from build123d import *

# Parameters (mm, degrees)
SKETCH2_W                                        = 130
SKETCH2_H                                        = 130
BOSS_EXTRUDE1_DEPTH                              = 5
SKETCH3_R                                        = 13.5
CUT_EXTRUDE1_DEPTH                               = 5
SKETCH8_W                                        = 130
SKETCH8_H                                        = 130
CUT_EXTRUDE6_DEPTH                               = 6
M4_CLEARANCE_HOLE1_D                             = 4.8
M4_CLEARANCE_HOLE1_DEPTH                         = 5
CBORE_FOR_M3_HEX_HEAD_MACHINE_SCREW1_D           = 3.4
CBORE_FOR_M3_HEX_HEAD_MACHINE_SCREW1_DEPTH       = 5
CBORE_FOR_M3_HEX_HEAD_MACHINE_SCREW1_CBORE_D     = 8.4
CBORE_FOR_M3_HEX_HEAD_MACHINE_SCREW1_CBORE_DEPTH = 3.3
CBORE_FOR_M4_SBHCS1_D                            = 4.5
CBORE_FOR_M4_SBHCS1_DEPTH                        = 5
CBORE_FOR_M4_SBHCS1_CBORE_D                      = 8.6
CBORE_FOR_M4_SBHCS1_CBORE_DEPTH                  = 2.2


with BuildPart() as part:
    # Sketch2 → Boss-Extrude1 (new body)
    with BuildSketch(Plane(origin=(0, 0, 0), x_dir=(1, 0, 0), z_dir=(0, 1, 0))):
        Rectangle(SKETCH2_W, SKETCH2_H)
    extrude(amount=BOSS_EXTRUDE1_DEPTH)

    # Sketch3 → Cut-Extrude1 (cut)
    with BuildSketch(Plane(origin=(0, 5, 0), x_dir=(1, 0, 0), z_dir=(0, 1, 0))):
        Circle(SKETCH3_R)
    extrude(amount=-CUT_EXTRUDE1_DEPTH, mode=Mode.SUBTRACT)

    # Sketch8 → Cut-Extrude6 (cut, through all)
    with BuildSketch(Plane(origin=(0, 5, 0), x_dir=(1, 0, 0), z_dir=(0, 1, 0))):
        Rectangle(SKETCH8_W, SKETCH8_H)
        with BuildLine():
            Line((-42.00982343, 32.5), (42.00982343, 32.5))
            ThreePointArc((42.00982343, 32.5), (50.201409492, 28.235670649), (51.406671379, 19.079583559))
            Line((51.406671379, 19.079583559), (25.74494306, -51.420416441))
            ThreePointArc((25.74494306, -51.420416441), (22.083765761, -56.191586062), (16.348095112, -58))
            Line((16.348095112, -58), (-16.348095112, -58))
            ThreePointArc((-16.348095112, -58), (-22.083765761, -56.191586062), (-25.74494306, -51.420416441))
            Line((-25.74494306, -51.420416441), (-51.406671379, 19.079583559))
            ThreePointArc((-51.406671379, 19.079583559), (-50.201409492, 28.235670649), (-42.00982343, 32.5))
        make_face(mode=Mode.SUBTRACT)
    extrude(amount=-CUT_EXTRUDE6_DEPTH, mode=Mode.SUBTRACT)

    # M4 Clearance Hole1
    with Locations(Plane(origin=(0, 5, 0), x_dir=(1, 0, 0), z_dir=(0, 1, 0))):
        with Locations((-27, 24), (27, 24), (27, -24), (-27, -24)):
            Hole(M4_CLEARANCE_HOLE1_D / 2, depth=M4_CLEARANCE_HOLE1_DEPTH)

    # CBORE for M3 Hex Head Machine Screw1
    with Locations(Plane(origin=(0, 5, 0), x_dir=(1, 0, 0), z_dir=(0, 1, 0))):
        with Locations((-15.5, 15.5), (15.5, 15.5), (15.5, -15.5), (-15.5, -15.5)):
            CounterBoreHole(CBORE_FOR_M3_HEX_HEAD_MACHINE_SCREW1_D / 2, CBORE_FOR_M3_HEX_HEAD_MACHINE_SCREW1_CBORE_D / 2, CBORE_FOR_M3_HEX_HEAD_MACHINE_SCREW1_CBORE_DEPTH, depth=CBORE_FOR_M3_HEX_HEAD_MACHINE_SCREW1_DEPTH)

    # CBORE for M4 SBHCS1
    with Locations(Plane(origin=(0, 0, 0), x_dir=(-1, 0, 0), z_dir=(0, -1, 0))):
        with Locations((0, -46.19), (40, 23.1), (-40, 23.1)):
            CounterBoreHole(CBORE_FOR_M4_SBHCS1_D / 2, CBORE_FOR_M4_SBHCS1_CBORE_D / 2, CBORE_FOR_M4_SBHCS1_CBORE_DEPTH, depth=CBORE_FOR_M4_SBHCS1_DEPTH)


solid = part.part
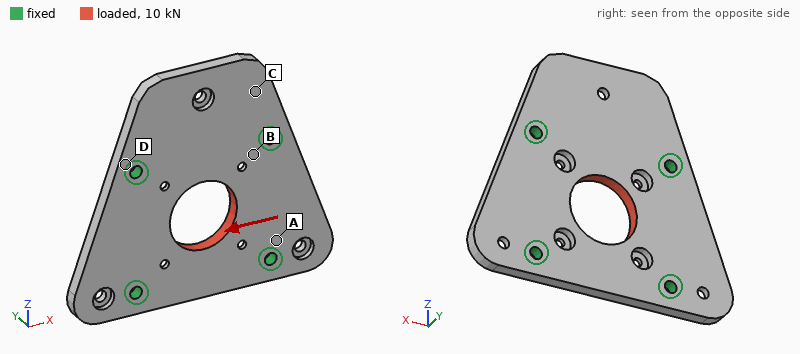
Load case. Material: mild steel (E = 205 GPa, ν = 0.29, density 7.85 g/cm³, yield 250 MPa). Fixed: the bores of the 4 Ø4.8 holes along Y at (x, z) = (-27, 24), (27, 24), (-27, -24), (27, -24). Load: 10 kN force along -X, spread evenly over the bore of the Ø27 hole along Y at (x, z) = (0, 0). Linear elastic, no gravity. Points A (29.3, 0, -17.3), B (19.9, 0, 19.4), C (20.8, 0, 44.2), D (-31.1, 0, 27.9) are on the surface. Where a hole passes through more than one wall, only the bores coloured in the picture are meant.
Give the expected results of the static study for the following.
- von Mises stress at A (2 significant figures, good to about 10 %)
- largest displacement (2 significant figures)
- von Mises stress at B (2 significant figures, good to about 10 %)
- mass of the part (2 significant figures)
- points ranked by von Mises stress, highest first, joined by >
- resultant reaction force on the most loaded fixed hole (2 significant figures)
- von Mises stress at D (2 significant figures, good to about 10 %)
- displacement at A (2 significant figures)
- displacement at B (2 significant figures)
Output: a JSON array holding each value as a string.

["23 MPa", "5.0 µm", "32 MPa", "240 g", "B > A > D > C", "2.6 kN", "12 MPa", "1.5 µm", "1.4 µm"]
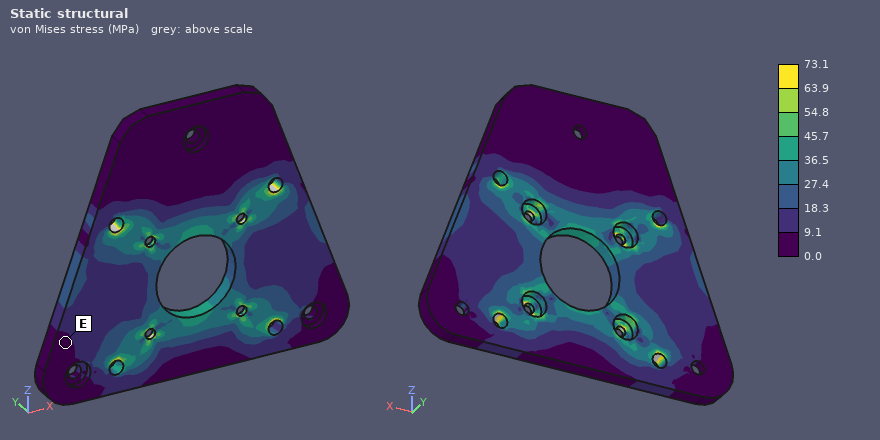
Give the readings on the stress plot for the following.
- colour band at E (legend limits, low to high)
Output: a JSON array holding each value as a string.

["0.0 to 9.1 MPa"]
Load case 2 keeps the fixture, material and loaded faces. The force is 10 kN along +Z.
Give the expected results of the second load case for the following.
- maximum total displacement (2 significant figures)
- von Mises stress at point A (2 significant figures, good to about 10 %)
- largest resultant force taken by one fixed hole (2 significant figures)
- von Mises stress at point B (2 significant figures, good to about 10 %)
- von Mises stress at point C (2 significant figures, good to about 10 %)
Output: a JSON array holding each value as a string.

["7.5 µm", "20 MPa", "2.7 kN", "29 MPa", "8.2 MPa"]
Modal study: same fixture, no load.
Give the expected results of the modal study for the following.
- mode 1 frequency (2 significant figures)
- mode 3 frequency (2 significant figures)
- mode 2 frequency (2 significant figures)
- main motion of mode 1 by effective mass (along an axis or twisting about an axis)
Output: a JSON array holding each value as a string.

["3200 Hz", "7100 Hz", "6800 Hz", "along Y"]
